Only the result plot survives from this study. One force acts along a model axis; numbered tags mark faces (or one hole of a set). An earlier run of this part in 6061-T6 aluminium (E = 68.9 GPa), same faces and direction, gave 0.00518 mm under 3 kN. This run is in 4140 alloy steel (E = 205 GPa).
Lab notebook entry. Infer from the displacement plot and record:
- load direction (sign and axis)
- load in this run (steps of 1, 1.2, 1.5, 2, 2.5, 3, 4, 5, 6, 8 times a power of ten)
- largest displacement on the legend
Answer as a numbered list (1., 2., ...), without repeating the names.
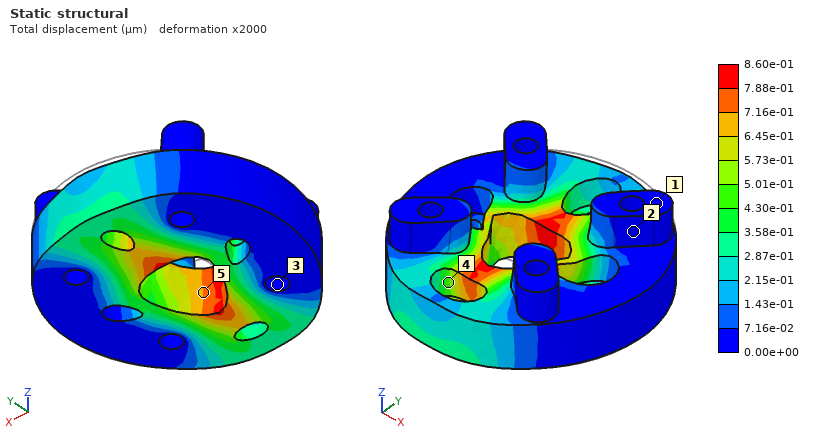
1. -Y
2. 1.5 kN
3. 8.60e-01 µm
